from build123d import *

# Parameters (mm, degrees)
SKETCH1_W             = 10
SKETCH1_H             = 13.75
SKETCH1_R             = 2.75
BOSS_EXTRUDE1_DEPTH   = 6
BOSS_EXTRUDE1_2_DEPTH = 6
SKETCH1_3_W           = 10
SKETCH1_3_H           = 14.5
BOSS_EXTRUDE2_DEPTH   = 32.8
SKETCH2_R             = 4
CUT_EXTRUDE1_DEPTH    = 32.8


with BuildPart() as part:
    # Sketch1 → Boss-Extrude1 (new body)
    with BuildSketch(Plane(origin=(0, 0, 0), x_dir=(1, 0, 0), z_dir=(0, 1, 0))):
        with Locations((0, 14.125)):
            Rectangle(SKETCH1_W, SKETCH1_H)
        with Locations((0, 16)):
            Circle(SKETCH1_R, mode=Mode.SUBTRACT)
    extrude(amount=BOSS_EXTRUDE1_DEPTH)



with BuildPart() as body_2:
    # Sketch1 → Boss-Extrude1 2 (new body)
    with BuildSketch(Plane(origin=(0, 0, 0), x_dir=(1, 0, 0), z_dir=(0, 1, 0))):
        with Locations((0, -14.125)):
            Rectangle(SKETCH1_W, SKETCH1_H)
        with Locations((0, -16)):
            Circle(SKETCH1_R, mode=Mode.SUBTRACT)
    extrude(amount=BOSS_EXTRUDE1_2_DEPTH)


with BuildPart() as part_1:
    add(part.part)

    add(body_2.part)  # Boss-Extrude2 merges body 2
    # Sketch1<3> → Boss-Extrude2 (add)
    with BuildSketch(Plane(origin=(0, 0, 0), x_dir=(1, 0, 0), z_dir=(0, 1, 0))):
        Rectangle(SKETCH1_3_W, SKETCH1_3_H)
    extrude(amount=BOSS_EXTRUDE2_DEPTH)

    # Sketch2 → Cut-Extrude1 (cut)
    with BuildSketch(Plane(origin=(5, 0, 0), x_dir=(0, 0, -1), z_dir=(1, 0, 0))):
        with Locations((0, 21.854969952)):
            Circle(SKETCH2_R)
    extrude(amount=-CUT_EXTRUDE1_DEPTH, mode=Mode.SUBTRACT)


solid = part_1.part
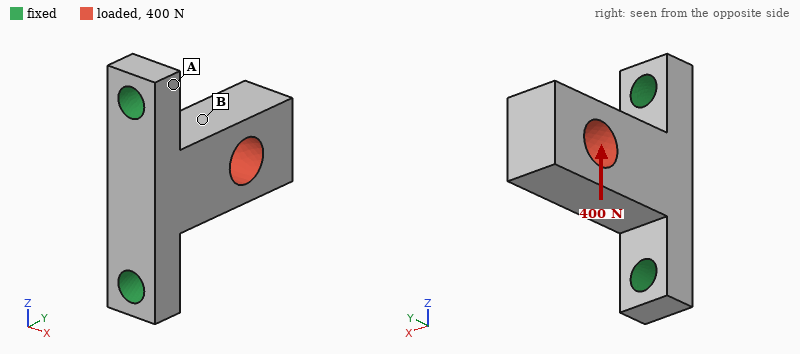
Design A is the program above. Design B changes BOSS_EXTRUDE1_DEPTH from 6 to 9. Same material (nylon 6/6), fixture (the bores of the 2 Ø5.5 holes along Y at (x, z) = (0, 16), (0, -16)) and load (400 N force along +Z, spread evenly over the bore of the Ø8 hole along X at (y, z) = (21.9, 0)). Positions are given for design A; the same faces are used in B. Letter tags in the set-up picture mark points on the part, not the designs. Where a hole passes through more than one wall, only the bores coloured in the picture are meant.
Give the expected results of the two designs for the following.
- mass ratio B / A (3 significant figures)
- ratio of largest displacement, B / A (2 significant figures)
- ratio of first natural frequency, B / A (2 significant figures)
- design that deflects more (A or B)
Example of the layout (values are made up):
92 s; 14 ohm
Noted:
1.06; 0.77; 1.2; A
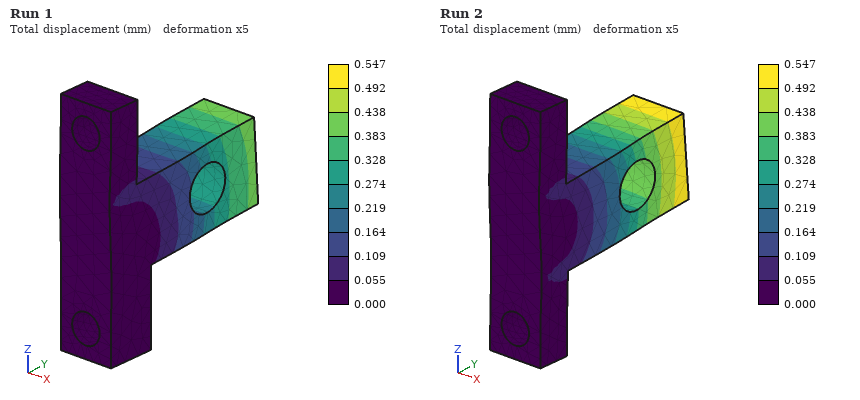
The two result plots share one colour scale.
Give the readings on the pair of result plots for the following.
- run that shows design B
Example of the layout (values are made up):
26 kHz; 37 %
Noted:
Run 1
